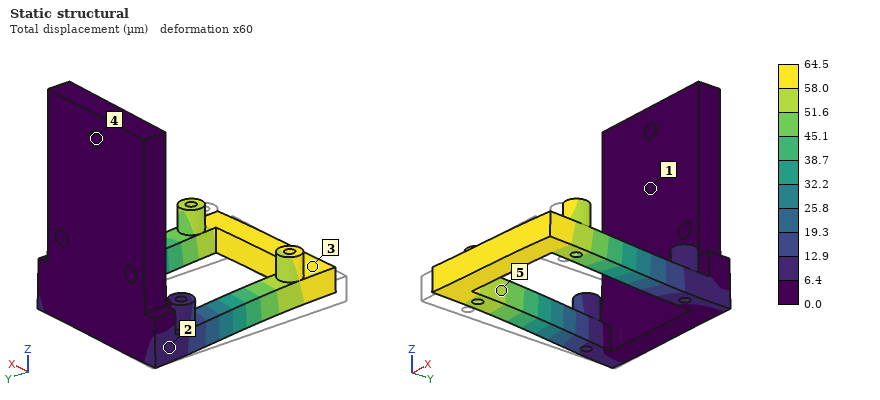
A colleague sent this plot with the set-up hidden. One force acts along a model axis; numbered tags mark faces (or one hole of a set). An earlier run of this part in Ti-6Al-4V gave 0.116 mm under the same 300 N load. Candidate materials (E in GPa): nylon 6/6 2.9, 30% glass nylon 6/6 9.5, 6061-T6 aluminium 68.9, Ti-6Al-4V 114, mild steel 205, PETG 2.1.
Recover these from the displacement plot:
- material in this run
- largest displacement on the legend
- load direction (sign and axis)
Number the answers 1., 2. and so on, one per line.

1. mild steel
2. 64.5 µm
3. +X
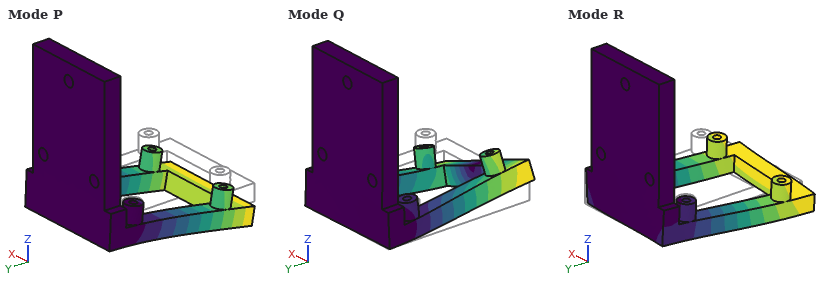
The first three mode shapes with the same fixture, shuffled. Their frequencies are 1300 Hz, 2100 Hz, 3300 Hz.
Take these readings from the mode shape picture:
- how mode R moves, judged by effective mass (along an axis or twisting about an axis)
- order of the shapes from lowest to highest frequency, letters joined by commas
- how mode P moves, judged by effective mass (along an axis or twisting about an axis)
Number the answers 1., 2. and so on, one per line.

1. along X
2. P, R, Q
3. along Z
